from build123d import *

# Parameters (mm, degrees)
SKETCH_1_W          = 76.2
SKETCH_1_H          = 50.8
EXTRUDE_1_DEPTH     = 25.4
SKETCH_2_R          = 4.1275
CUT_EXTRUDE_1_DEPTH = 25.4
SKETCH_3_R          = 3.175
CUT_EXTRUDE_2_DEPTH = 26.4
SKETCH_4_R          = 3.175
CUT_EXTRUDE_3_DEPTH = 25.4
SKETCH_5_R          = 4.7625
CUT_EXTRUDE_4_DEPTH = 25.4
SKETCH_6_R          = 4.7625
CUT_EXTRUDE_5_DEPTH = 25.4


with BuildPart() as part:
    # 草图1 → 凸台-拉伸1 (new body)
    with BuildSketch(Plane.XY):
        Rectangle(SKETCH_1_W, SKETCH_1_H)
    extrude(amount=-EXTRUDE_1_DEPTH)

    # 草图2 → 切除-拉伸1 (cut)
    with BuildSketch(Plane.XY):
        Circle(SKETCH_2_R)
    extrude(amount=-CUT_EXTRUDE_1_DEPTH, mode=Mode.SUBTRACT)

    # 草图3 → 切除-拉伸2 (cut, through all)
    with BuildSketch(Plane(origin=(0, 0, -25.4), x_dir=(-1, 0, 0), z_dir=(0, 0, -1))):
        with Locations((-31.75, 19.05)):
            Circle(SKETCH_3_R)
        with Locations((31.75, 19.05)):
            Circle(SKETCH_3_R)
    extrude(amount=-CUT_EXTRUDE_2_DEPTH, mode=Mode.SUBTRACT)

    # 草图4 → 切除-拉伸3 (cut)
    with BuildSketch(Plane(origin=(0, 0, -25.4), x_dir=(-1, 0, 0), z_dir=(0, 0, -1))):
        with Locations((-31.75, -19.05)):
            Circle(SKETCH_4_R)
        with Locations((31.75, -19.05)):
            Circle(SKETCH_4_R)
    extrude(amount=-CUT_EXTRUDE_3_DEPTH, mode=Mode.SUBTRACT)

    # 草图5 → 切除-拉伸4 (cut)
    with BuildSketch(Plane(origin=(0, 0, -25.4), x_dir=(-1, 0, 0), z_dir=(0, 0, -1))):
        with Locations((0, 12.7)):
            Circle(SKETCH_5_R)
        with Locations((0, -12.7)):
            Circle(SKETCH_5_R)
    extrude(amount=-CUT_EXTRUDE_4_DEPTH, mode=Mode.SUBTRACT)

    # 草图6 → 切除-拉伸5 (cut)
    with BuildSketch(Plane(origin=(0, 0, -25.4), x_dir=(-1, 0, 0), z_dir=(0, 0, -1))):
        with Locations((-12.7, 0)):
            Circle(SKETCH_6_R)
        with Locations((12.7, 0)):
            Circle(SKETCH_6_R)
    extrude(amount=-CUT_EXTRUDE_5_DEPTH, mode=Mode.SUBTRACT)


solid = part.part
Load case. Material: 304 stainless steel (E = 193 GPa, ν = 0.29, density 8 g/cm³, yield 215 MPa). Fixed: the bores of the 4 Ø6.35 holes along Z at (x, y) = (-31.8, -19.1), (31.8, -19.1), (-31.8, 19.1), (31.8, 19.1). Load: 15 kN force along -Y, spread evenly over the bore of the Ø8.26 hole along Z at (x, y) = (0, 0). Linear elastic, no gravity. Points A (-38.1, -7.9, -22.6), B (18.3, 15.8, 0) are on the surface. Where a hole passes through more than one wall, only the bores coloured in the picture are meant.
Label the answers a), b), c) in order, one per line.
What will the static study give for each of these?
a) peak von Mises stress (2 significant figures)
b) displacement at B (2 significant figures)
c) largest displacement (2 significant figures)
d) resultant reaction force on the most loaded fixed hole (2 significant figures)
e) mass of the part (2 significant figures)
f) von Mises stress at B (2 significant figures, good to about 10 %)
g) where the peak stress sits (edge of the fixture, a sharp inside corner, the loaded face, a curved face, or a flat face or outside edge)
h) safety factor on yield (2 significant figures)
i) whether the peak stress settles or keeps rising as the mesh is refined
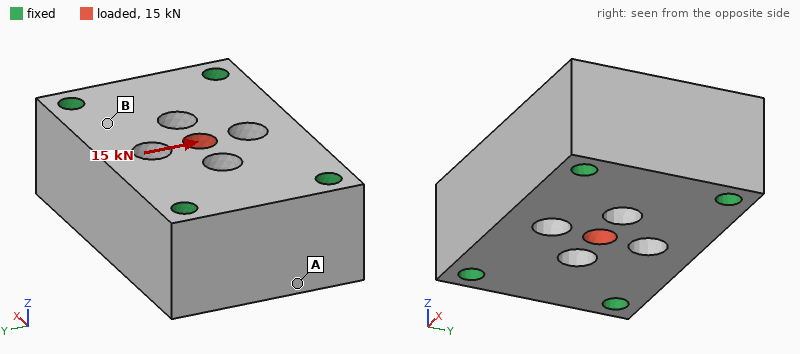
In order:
a) 51 MPa
b) 1.5 µm
c) 4.9 µm
d) 4.9 kN
e) 690 g
f) 16 MPa
g) the loaded face
h) 4.2
i) settles
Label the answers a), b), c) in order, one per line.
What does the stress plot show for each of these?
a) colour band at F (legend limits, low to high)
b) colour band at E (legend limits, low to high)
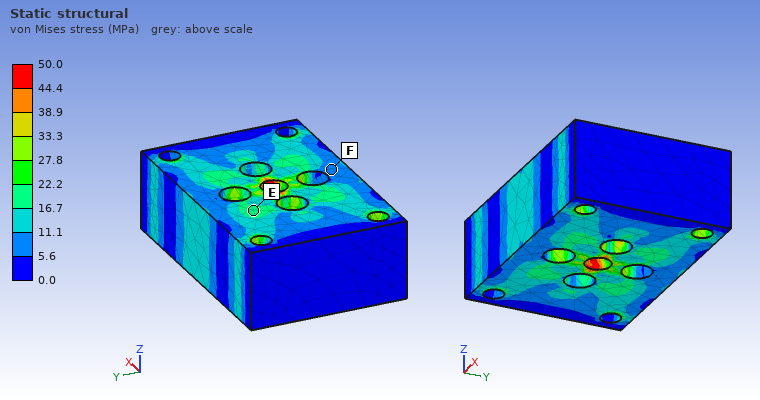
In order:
a) 5.6 to 11.1 MPa
b) 16.7 to 22.2 MPa
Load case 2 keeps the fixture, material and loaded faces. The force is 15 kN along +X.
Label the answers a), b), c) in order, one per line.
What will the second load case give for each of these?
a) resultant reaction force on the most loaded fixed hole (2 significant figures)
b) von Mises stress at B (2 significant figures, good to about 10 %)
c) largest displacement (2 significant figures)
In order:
a) 4.0 kN
b) 11 MPa
c) 3.3 µm
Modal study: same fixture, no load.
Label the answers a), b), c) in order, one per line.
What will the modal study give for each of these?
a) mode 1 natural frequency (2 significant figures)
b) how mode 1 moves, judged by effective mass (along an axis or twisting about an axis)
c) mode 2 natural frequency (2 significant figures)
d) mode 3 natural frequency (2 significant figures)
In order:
a) 17 kHz
b) along Z
c) 22 kHz
d) 22 kHz
